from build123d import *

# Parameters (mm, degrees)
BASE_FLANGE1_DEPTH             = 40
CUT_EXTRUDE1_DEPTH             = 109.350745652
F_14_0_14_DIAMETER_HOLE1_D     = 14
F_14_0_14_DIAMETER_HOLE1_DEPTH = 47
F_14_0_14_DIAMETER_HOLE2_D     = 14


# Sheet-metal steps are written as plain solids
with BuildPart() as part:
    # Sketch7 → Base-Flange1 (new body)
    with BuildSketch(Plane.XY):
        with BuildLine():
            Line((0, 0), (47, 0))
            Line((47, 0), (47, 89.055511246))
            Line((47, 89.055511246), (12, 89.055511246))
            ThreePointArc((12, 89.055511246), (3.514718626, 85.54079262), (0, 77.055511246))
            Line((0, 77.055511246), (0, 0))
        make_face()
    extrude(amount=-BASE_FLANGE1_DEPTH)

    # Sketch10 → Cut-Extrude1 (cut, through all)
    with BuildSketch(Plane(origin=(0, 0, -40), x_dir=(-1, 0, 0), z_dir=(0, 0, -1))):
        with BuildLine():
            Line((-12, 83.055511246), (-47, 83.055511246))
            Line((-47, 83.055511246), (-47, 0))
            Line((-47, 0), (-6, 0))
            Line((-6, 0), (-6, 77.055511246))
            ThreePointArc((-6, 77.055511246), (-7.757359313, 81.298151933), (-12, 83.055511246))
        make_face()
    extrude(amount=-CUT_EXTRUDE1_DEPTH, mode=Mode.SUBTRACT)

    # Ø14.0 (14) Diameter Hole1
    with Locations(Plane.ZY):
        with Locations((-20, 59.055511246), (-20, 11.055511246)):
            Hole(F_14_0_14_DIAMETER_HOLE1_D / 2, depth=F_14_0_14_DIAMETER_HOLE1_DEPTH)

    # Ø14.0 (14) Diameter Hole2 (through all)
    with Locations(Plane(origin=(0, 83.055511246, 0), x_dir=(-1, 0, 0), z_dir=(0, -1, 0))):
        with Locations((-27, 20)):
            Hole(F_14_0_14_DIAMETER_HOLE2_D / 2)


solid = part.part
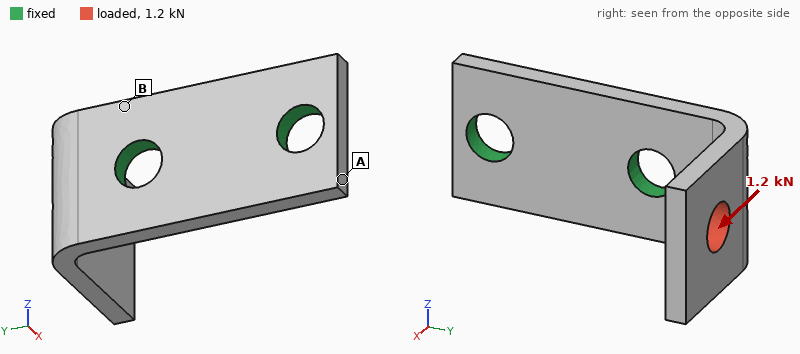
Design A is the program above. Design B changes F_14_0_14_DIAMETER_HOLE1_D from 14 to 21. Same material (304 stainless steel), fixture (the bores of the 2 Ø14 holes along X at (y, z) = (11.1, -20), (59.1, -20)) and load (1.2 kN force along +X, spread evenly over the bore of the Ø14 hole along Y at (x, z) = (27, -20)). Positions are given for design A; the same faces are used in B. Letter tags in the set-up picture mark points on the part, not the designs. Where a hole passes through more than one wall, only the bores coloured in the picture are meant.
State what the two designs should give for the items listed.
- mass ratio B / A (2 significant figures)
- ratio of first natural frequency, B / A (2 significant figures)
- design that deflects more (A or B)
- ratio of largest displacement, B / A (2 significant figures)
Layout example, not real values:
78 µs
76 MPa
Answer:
0.92
1.1
A
0.68
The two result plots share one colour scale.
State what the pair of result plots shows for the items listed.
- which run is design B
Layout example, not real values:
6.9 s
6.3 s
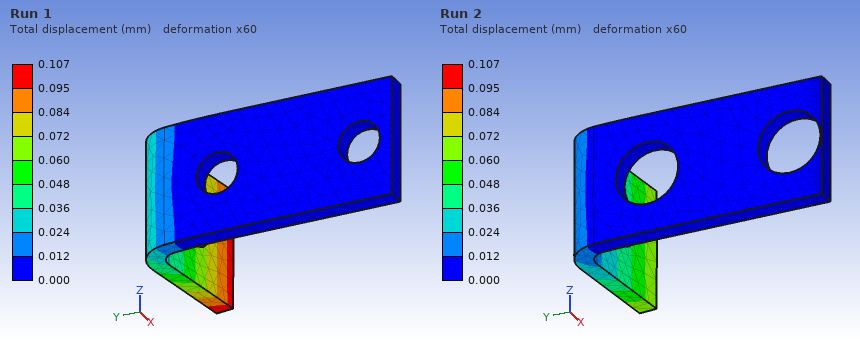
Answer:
Run 2
